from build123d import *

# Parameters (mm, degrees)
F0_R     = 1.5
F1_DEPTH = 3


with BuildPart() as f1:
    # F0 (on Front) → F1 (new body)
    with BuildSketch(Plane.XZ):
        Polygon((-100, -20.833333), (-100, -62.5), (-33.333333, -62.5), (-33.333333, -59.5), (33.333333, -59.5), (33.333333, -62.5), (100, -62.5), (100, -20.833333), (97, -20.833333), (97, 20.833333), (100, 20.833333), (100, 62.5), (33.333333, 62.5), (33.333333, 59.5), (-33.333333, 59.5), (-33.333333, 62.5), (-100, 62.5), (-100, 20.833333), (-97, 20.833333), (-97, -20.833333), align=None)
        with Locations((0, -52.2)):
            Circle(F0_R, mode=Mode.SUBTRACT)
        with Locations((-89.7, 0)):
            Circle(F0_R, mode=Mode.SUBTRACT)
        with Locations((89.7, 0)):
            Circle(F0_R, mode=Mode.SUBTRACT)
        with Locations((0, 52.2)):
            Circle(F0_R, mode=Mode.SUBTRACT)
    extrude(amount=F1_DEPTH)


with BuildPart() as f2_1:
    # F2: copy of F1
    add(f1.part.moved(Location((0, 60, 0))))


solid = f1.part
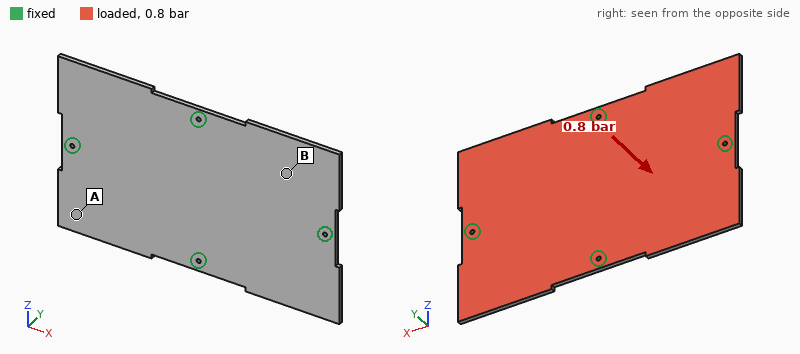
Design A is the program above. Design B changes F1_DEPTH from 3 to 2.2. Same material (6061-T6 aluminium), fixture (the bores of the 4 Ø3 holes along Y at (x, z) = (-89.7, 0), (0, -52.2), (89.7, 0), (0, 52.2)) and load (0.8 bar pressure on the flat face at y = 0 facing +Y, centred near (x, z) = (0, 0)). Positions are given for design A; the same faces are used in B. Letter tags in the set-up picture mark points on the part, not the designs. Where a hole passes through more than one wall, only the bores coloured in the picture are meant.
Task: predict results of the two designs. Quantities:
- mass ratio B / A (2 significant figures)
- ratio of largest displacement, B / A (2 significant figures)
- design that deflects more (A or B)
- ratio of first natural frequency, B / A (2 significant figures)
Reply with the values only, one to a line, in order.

0.73
2.5
B
0.75
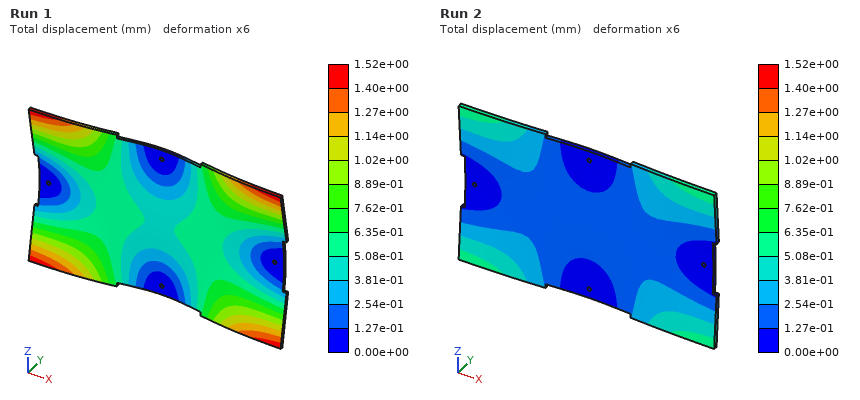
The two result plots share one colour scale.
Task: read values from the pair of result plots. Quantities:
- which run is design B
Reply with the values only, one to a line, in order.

Run 1
